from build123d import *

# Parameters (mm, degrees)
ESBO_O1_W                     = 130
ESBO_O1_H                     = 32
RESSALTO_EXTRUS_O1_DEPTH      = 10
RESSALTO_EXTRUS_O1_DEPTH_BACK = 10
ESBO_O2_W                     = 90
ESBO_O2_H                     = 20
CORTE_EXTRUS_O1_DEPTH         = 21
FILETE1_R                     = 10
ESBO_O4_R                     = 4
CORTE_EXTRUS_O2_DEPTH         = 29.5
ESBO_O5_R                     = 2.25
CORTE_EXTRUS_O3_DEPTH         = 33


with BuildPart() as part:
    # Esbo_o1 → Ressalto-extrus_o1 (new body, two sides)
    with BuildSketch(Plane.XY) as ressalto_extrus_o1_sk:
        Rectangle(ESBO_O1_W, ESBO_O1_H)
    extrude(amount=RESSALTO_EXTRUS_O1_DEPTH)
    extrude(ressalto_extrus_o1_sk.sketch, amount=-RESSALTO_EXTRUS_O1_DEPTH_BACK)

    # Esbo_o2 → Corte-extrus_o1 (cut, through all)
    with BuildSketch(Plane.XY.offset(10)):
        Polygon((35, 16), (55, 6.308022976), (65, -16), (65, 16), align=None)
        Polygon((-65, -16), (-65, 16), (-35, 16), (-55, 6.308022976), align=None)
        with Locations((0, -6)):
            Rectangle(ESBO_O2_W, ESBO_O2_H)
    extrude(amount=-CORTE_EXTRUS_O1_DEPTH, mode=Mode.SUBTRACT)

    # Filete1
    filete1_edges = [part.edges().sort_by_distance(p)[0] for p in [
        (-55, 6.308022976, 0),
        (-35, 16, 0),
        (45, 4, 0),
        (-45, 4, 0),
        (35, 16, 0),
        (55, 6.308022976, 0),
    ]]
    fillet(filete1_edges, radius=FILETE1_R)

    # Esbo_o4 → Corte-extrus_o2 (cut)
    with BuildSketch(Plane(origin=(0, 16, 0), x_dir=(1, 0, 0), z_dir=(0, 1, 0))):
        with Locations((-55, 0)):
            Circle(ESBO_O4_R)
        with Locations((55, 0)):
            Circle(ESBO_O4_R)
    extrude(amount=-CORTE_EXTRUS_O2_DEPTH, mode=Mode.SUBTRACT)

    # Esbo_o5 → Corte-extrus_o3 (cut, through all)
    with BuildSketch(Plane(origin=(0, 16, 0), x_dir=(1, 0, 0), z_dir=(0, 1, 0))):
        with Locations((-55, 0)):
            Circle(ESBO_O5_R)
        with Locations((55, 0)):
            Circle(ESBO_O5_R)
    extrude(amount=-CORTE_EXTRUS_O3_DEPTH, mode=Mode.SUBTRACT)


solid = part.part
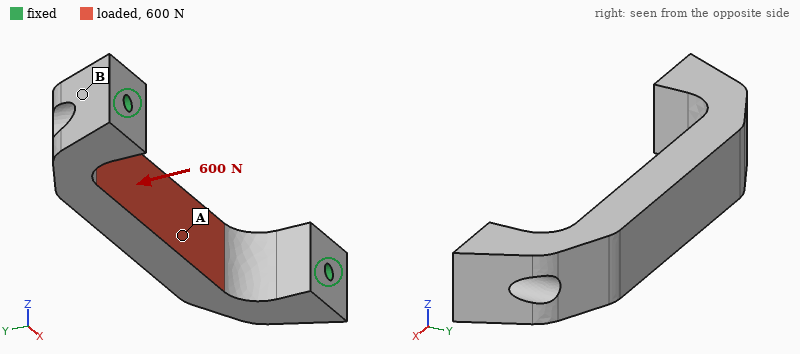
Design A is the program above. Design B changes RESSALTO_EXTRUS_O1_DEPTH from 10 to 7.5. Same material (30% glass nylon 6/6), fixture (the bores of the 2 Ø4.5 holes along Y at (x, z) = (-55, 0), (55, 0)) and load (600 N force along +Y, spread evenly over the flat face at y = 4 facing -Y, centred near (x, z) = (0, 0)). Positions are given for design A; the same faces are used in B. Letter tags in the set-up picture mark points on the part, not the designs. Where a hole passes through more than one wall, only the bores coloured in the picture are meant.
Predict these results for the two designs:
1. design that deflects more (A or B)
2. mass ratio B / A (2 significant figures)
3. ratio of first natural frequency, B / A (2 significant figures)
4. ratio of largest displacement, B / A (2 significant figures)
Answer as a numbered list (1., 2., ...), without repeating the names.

1. B
2. 0.87
3. 1.1
4. 1.3
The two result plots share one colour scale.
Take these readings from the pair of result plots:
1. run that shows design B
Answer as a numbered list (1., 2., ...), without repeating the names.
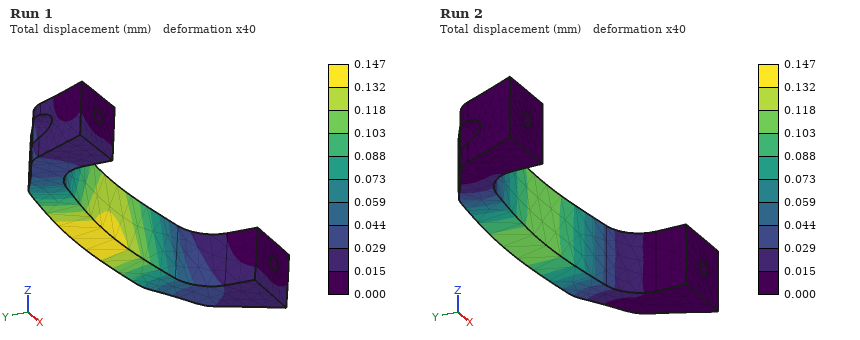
1. Run 1
